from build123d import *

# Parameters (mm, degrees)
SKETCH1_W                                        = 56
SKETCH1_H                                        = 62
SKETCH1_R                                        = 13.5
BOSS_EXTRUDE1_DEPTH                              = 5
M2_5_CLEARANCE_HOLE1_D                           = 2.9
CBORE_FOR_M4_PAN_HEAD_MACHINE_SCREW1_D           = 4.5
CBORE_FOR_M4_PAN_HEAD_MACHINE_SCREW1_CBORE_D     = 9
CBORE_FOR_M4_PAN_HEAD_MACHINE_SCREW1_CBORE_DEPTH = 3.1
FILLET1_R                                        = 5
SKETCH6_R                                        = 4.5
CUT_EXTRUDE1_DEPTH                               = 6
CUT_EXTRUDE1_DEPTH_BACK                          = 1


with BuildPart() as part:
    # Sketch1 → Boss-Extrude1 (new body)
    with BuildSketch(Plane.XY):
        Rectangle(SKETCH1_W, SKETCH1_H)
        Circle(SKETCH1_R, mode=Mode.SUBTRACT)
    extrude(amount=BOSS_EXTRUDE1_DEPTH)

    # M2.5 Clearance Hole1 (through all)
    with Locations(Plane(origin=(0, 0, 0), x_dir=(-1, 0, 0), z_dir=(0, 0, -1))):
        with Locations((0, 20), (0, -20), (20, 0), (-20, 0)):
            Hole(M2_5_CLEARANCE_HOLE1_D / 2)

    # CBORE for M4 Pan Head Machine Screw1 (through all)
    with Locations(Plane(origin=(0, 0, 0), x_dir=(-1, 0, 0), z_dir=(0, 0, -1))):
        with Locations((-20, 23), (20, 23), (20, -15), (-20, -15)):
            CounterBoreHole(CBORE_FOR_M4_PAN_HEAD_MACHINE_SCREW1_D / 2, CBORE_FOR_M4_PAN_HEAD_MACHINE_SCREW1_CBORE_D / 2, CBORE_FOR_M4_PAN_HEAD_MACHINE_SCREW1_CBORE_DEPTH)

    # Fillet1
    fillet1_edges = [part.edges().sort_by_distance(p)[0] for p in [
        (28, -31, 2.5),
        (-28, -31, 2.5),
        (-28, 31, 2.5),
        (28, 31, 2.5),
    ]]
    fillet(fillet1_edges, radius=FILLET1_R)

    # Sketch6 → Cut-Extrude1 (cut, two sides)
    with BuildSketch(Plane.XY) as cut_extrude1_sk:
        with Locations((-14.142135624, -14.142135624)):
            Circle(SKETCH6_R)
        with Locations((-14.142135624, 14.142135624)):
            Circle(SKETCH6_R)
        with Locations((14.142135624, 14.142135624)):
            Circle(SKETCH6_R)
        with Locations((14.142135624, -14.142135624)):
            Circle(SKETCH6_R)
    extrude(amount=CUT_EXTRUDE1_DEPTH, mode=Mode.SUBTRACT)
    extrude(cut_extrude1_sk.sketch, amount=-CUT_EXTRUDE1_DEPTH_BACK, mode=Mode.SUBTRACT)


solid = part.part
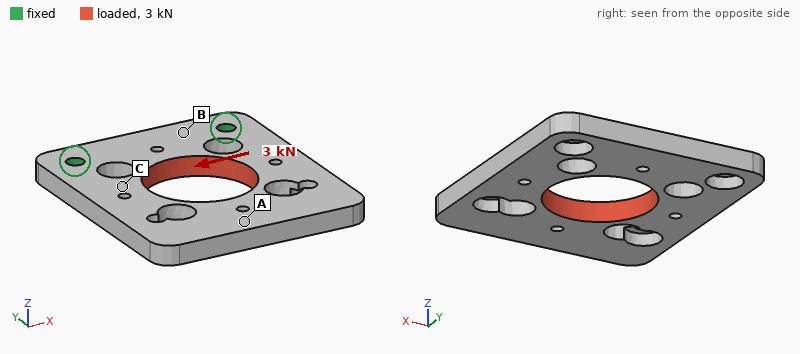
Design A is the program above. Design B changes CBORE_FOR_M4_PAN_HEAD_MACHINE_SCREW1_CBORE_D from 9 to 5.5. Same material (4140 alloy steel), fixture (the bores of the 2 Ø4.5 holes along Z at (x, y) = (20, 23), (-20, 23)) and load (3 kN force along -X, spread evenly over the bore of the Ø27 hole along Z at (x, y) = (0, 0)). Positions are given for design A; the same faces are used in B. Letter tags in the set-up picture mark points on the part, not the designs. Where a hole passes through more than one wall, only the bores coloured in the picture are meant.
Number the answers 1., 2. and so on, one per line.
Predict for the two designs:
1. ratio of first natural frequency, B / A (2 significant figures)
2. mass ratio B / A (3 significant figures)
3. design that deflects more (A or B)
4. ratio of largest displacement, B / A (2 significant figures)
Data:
1. 1.1
2. 1.04
3. A
4. 0.87
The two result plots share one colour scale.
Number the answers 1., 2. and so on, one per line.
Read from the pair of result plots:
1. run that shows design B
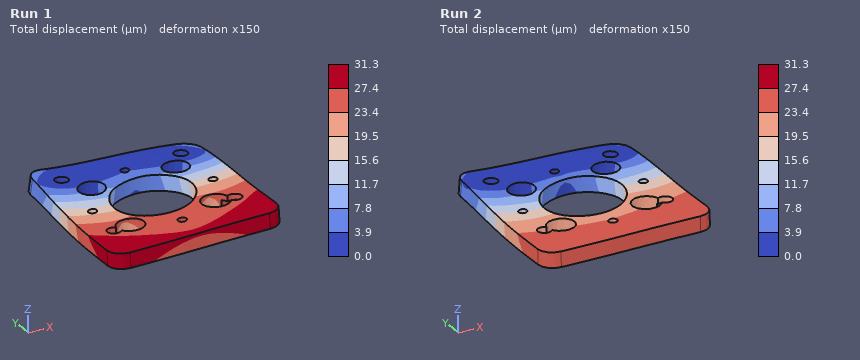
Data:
1. Run 2
